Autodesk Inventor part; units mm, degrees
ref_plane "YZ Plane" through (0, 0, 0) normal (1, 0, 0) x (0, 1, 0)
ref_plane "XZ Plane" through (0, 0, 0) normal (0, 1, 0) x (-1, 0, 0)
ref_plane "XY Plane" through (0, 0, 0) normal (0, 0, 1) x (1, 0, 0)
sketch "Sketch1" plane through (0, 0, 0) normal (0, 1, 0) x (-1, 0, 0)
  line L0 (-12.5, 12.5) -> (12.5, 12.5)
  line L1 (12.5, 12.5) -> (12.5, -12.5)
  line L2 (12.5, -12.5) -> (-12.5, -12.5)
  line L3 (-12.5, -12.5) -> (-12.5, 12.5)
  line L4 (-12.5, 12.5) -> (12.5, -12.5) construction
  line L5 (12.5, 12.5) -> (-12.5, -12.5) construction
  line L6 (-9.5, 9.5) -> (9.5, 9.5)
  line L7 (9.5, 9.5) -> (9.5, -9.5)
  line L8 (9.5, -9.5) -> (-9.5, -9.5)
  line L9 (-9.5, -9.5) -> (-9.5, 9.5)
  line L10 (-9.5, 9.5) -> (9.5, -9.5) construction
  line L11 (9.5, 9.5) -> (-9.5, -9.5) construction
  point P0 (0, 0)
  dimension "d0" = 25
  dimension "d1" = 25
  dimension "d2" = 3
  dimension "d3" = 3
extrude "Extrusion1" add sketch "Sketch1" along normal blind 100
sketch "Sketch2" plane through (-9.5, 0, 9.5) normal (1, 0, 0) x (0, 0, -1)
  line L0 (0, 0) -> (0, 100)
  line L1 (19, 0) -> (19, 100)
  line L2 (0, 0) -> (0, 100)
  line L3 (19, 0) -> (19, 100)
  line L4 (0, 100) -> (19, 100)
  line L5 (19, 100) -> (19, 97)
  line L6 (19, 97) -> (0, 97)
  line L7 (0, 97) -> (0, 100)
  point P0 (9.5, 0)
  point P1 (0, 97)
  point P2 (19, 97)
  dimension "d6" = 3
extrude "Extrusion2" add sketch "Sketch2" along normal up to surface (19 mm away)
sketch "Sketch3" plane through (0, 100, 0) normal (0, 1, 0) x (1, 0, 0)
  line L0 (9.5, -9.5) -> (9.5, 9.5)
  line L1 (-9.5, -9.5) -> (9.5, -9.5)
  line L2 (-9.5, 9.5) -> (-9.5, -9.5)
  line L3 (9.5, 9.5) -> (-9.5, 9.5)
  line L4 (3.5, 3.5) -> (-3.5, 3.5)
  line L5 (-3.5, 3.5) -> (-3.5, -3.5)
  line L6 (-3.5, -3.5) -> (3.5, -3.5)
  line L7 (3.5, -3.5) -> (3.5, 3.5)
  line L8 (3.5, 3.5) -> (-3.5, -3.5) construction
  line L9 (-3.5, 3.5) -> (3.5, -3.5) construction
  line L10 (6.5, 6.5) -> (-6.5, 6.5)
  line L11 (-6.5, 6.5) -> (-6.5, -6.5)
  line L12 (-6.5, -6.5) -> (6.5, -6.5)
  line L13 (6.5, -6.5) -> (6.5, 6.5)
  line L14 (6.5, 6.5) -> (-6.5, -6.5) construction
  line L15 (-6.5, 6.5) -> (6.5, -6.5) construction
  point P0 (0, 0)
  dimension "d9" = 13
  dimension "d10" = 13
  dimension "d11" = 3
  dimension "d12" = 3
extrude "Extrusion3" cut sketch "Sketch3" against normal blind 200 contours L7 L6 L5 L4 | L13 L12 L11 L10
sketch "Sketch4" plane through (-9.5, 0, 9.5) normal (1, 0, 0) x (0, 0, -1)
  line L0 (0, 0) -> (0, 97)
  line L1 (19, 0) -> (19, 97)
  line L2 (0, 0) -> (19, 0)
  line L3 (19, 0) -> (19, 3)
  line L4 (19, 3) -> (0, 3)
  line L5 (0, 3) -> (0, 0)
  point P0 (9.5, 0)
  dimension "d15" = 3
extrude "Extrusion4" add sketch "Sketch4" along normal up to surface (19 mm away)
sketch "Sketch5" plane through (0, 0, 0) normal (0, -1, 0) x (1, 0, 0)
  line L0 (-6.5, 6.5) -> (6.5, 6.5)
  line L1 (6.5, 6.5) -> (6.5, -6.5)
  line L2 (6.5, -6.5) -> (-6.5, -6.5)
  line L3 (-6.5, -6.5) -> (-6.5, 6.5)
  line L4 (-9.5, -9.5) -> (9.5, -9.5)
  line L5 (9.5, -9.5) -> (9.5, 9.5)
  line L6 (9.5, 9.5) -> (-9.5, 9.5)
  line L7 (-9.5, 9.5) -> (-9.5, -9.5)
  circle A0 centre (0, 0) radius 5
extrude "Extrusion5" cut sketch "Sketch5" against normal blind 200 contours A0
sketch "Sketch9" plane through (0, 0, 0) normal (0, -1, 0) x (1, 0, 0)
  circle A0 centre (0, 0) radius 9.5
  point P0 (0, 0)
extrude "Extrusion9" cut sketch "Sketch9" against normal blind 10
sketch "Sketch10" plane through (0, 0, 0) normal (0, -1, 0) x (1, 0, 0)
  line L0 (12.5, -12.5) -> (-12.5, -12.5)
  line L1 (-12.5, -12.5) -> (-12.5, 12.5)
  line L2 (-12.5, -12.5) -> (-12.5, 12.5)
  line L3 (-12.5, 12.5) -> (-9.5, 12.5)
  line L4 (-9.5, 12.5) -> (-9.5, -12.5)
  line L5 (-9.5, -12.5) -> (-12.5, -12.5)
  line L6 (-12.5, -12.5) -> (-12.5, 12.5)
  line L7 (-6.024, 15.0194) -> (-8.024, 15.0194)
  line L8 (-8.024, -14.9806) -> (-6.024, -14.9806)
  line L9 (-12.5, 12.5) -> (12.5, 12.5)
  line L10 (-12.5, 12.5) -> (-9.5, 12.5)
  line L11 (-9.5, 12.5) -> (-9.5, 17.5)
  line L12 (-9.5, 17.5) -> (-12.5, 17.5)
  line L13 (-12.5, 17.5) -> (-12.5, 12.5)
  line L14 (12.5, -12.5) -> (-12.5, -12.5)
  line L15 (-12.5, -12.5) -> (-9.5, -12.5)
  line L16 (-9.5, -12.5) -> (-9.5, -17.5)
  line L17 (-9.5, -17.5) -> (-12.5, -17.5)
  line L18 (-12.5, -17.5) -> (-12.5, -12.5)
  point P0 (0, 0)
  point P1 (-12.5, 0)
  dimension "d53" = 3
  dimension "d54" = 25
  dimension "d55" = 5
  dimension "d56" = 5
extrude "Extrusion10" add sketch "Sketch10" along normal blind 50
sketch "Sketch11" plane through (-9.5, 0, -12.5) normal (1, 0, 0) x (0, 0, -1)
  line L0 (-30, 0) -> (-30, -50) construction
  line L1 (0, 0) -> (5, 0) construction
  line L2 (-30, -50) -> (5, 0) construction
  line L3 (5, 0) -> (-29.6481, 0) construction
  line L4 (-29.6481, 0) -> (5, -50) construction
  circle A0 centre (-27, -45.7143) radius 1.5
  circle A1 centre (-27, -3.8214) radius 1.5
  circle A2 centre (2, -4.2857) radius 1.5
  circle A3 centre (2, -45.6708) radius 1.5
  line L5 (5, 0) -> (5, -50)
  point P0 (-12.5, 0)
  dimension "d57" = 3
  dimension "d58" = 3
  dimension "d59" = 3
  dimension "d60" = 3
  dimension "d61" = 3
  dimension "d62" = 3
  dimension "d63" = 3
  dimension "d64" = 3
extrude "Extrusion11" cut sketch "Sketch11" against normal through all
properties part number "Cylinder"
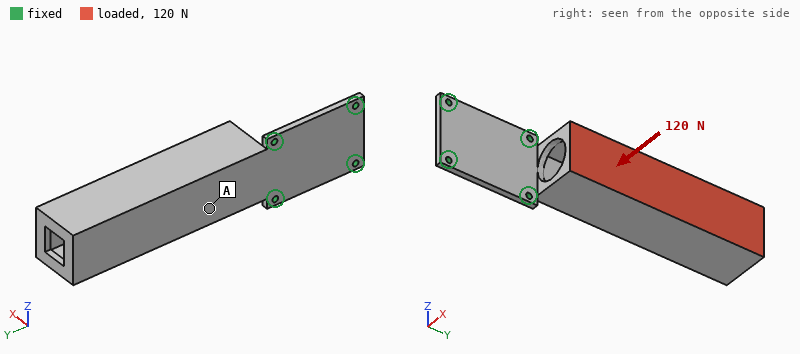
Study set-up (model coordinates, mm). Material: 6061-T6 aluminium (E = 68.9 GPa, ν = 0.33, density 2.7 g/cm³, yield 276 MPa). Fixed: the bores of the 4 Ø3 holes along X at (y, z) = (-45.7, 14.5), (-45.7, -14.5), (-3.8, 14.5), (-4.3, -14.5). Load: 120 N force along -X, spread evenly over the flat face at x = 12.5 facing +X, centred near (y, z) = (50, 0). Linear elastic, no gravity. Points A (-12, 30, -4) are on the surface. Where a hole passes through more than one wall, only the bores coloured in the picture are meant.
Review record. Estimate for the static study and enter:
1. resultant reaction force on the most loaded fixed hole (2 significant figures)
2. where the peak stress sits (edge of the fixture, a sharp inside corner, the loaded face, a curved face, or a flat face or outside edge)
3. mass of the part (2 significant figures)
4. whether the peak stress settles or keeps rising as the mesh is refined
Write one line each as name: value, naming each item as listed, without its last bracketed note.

resultant reaction force on the most loaded fixed hole: 99 N
where the peak stress sits: edge of the fixture
mass of the part: 87 g
whether the peak stress settles or keeps rising as the mesh is refined: keeps rising
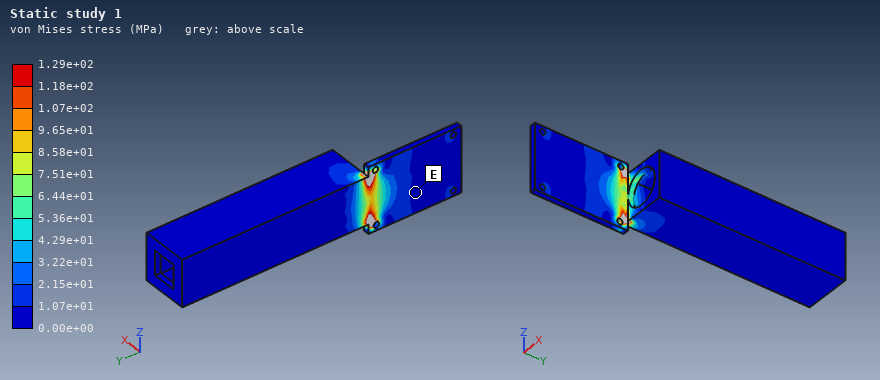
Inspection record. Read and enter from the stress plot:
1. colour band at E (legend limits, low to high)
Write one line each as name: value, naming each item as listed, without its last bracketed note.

colour band at E: 0.00e+00 to 1.07e+01 MPa
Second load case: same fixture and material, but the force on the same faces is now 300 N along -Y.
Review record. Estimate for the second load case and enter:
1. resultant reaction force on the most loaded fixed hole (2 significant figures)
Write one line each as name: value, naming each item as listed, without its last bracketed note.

resultant reaction force on the most loaded fixed hole: 130 N
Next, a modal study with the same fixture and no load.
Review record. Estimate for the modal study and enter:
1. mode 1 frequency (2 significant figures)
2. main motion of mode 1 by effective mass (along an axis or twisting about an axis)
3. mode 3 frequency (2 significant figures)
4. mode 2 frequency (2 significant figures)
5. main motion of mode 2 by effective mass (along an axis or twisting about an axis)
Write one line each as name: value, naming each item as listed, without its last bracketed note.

mode 1 frequency: 210 Hz
main motion of mode 1 by effective mass: along X
mode 3 frequency: 2500 Hz
mode 2 frequency: 1200 Hz
main motion of mode 2 by effective mass: along Z
